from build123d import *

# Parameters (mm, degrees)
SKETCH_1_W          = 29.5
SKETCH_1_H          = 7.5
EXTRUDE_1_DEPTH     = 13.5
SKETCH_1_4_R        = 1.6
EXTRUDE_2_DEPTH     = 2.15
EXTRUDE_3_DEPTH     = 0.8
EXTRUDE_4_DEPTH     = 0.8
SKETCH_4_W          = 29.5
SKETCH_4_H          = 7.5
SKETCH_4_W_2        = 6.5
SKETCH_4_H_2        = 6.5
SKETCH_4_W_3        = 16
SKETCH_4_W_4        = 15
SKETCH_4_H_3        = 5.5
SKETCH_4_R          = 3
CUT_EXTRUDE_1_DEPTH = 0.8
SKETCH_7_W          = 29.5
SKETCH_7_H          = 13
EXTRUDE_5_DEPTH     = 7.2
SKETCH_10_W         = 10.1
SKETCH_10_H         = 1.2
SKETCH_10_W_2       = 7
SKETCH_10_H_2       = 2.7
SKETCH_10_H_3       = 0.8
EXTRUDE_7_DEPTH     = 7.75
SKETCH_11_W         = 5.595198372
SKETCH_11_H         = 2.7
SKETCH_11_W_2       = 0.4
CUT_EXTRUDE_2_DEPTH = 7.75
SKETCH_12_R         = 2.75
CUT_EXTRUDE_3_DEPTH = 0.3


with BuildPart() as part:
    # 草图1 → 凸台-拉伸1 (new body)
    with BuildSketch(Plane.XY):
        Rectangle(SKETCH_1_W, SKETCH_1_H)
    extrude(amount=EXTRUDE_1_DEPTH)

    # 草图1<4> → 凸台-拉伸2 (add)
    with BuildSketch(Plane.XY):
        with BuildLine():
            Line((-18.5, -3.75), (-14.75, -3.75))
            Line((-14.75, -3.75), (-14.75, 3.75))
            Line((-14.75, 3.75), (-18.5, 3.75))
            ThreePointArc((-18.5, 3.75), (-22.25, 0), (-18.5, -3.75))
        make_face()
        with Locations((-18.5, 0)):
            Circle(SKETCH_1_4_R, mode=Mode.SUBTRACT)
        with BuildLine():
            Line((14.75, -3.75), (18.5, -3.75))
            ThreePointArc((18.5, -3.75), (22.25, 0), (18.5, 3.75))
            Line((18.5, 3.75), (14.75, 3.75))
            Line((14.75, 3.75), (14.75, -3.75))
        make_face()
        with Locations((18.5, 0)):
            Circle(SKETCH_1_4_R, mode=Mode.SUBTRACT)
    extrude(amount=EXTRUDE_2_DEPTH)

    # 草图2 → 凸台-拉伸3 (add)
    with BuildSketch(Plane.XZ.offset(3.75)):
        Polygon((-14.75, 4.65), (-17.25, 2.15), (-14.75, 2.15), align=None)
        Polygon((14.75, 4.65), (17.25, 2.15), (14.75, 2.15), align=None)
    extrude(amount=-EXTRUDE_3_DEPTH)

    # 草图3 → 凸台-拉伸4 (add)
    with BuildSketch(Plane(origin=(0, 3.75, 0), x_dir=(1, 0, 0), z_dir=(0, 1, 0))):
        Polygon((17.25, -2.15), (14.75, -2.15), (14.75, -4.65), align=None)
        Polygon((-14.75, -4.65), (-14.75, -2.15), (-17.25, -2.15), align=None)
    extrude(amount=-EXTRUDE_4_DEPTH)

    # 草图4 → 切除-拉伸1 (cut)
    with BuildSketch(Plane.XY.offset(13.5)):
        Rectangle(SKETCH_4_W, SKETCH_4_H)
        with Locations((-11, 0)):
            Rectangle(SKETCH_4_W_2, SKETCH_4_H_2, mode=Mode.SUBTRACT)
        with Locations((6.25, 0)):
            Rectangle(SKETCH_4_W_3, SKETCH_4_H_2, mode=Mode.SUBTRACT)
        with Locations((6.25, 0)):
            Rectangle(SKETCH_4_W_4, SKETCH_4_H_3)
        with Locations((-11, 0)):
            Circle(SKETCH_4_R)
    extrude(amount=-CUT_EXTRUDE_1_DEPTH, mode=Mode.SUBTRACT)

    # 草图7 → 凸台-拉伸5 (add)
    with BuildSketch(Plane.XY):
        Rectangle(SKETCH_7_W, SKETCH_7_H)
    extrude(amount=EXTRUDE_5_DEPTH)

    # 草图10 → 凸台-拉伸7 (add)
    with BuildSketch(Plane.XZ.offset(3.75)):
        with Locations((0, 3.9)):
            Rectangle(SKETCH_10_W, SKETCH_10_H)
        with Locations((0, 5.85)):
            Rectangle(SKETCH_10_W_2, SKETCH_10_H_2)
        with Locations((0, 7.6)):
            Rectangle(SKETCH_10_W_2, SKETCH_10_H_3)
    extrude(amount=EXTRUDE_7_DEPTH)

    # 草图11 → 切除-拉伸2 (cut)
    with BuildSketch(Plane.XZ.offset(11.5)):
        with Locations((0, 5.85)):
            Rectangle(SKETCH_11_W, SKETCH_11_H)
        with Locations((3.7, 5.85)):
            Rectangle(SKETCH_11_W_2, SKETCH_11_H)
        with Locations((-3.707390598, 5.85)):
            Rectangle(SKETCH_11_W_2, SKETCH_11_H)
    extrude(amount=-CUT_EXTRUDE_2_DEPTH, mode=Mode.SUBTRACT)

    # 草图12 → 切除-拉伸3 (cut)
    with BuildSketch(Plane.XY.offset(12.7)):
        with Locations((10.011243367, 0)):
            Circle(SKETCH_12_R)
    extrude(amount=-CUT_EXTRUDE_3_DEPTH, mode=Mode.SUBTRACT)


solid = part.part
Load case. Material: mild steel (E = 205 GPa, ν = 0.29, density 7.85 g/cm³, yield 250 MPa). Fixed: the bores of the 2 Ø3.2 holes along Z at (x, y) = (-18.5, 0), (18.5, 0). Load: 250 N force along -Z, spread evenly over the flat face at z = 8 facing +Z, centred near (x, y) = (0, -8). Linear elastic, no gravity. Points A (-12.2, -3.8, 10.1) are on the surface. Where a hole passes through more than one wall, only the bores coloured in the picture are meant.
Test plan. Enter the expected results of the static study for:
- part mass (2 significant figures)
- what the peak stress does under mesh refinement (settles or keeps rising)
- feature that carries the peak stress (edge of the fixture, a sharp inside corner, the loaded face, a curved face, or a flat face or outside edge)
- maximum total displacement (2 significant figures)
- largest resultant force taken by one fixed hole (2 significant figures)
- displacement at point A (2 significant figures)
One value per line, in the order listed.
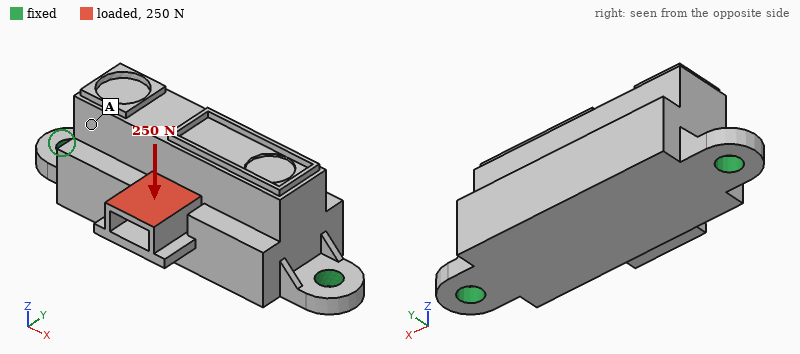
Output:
33 g
keeps rising
edge of the fixture
21 µm
170 N
10 µm
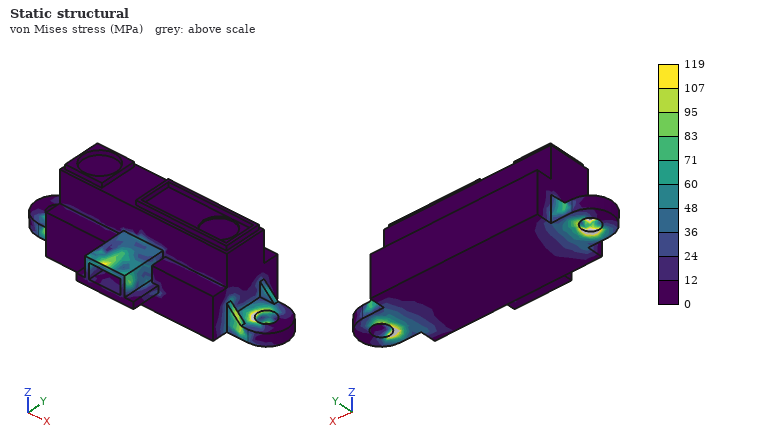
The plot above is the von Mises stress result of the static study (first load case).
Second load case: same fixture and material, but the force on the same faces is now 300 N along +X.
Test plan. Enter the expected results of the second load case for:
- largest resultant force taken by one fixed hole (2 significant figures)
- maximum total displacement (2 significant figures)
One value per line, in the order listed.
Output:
180 N
5.4 µm
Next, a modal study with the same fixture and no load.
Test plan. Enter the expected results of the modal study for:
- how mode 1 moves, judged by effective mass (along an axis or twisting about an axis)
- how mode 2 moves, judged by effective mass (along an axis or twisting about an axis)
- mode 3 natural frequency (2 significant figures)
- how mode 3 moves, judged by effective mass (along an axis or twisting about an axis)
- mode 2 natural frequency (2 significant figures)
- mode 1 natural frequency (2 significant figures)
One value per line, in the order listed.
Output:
along Y
along Z
20 kHz
along Y
14 kHz
5500 Hz
